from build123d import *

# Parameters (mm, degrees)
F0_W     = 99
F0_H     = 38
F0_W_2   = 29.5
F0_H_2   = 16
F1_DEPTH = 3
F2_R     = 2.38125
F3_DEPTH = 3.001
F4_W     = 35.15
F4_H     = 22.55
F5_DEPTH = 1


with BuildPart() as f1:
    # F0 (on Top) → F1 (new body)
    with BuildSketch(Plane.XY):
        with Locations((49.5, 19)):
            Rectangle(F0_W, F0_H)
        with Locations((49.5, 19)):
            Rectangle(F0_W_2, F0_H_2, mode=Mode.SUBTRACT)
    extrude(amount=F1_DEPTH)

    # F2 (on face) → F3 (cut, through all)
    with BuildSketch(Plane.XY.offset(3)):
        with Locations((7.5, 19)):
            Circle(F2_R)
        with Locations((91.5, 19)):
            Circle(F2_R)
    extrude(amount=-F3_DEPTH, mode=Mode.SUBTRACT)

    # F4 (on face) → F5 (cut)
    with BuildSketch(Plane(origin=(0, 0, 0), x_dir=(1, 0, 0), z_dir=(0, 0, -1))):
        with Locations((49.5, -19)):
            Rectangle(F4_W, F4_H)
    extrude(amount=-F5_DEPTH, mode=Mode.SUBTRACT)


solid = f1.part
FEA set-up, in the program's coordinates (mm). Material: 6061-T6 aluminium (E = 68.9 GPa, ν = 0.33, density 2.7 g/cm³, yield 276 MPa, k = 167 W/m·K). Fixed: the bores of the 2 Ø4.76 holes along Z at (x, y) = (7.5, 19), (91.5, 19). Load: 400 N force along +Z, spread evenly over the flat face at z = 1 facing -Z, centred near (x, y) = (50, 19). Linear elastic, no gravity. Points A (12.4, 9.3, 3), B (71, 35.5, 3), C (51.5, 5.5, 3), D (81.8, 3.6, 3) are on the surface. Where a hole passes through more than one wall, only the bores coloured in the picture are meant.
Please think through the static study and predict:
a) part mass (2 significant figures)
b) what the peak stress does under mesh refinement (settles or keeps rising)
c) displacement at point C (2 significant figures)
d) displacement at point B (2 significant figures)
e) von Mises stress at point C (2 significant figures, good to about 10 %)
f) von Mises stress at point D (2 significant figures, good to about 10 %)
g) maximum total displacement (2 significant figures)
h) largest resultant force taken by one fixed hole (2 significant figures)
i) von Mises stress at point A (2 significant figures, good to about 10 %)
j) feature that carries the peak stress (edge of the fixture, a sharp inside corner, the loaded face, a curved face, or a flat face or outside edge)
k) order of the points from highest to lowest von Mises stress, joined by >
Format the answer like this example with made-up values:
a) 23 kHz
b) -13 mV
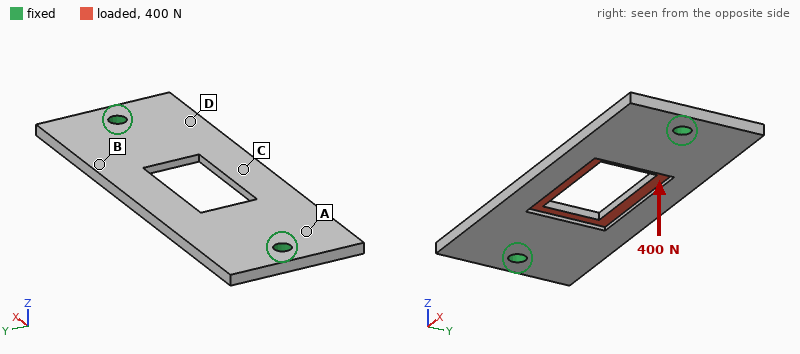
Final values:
a) 25 g
b) keeps rising
c) 0.25 mm
d) 0.13 mm
e) 64 MPa
f) 33 MPa
g) 0.27 mm
h) 230 N
i) 46 MPa
j) edge of the fixture
k) C > A > D > B
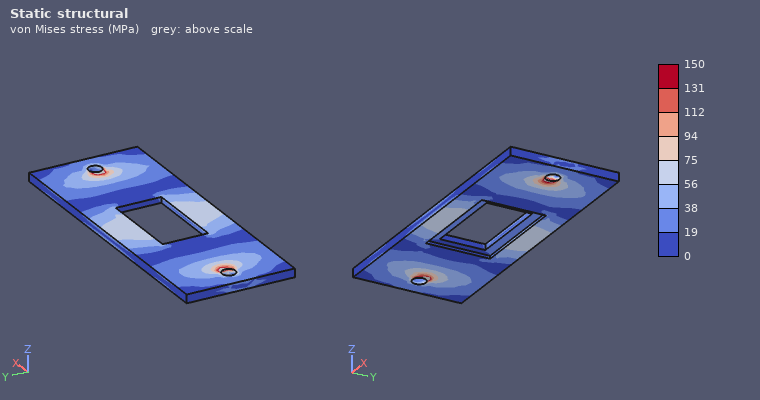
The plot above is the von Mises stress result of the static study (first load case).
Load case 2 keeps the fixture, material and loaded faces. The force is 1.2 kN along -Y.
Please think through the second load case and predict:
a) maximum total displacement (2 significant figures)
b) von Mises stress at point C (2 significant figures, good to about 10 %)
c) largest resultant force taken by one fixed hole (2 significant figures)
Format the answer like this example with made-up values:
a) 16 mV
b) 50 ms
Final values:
a) 37 µm
b) 19 MPa
c) 600 N
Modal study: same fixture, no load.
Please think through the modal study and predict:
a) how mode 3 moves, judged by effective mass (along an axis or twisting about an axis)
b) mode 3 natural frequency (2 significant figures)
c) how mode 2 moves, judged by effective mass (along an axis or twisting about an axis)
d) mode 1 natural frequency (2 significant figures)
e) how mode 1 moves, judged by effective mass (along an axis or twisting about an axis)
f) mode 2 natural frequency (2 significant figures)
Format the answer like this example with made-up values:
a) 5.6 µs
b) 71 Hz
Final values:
a) twisting about Y
b) 4900 Hz
c) twisting about X
d) 2300 Hz
e) along Z
f) 2700 Hz
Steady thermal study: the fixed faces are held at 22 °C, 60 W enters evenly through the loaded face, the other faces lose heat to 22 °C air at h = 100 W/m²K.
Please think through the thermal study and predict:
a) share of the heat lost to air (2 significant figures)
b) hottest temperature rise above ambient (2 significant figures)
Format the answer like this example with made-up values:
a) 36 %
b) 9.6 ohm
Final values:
a) 30 %
b) 56 K
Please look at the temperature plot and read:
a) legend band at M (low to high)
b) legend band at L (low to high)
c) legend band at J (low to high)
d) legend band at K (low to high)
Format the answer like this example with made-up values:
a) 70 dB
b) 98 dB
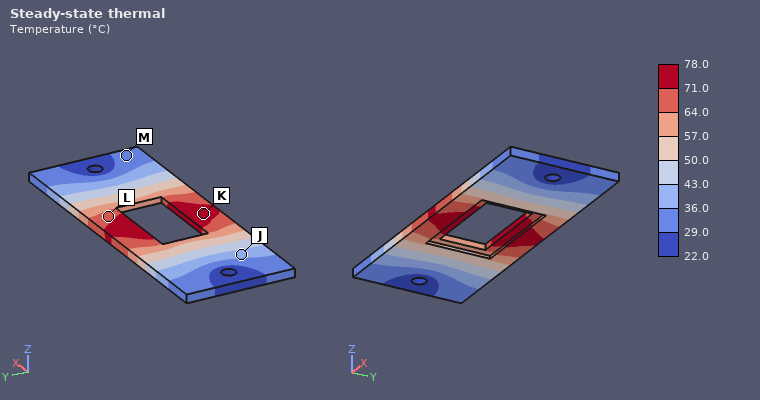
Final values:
a) 29.0 to 36.0 °C
b) 64.0 to 71.0 °C
c) 36.0 to 43.0 °C
d) 71.0 to 78.0 °C
